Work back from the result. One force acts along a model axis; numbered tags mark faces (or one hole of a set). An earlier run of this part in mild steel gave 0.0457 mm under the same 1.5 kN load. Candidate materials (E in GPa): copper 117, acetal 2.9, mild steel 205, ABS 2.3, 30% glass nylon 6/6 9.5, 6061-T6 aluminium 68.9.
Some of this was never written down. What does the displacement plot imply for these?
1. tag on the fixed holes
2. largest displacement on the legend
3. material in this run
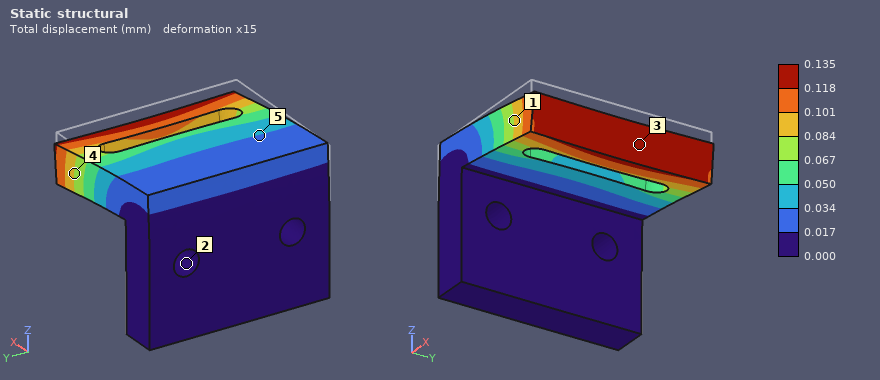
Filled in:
2
0.135 mm
6061-T6 aluminium
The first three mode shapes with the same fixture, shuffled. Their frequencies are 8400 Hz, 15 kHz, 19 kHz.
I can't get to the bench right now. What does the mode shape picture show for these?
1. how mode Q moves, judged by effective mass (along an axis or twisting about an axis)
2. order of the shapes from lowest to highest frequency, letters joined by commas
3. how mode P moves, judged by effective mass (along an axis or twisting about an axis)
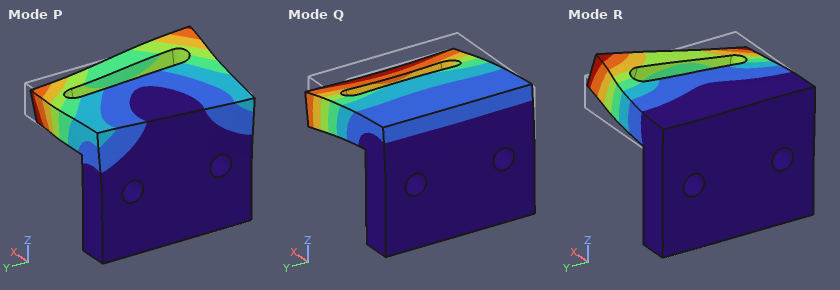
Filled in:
along Z
Q, P, R
along Y
